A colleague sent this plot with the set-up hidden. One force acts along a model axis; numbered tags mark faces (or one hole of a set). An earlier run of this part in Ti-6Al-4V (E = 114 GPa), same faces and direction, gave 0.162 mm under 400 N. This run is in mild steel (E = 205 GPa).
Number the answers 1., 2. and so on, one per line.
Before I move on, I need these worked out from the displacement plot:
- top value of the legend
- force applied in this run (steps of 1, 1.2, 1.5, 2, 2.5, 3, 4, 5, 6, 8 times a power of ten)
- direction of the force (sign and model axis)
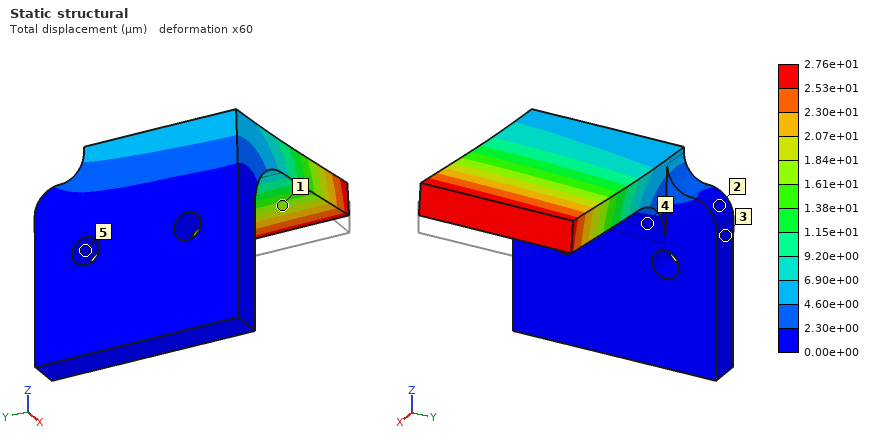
1. 2.76e+01 µm
2. 120 N
3. +Z
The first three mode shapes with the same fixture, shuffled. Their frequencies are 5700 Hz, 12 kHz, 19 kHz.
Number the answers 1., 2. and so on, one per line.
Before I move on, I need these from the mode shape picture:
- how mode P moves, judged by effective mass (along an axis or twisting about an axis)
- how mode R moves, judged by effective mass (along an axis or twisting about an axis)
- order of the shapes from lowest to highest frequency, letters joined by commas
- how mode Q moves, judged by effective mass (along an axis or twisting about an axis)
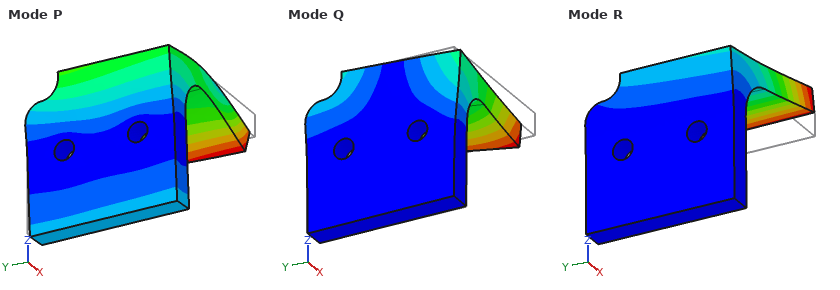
1. along X
2. along Z
3. R, Q, P
4. along Y
